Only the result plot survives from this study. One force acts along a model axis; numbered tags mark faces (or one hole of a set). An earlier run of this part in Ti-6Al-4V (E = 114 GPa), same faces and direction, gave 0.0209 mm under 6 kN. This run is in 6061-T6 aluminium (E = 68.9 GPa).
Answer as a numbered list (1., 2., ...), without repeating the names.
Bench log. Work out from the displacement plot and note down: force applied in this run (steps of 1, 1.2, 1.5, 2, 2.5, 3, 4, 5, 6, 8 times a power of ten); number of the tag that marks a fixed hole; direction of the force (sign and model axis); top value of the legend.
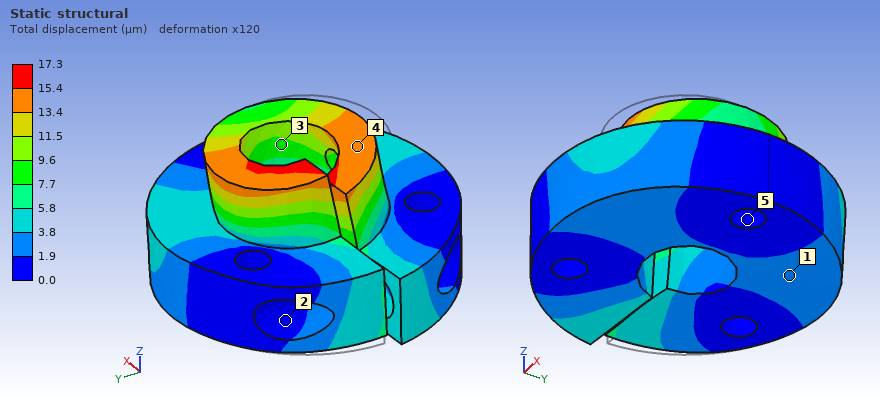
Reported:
1. 3 kN
2. 5
3. +Y
4. 17.3 µm
